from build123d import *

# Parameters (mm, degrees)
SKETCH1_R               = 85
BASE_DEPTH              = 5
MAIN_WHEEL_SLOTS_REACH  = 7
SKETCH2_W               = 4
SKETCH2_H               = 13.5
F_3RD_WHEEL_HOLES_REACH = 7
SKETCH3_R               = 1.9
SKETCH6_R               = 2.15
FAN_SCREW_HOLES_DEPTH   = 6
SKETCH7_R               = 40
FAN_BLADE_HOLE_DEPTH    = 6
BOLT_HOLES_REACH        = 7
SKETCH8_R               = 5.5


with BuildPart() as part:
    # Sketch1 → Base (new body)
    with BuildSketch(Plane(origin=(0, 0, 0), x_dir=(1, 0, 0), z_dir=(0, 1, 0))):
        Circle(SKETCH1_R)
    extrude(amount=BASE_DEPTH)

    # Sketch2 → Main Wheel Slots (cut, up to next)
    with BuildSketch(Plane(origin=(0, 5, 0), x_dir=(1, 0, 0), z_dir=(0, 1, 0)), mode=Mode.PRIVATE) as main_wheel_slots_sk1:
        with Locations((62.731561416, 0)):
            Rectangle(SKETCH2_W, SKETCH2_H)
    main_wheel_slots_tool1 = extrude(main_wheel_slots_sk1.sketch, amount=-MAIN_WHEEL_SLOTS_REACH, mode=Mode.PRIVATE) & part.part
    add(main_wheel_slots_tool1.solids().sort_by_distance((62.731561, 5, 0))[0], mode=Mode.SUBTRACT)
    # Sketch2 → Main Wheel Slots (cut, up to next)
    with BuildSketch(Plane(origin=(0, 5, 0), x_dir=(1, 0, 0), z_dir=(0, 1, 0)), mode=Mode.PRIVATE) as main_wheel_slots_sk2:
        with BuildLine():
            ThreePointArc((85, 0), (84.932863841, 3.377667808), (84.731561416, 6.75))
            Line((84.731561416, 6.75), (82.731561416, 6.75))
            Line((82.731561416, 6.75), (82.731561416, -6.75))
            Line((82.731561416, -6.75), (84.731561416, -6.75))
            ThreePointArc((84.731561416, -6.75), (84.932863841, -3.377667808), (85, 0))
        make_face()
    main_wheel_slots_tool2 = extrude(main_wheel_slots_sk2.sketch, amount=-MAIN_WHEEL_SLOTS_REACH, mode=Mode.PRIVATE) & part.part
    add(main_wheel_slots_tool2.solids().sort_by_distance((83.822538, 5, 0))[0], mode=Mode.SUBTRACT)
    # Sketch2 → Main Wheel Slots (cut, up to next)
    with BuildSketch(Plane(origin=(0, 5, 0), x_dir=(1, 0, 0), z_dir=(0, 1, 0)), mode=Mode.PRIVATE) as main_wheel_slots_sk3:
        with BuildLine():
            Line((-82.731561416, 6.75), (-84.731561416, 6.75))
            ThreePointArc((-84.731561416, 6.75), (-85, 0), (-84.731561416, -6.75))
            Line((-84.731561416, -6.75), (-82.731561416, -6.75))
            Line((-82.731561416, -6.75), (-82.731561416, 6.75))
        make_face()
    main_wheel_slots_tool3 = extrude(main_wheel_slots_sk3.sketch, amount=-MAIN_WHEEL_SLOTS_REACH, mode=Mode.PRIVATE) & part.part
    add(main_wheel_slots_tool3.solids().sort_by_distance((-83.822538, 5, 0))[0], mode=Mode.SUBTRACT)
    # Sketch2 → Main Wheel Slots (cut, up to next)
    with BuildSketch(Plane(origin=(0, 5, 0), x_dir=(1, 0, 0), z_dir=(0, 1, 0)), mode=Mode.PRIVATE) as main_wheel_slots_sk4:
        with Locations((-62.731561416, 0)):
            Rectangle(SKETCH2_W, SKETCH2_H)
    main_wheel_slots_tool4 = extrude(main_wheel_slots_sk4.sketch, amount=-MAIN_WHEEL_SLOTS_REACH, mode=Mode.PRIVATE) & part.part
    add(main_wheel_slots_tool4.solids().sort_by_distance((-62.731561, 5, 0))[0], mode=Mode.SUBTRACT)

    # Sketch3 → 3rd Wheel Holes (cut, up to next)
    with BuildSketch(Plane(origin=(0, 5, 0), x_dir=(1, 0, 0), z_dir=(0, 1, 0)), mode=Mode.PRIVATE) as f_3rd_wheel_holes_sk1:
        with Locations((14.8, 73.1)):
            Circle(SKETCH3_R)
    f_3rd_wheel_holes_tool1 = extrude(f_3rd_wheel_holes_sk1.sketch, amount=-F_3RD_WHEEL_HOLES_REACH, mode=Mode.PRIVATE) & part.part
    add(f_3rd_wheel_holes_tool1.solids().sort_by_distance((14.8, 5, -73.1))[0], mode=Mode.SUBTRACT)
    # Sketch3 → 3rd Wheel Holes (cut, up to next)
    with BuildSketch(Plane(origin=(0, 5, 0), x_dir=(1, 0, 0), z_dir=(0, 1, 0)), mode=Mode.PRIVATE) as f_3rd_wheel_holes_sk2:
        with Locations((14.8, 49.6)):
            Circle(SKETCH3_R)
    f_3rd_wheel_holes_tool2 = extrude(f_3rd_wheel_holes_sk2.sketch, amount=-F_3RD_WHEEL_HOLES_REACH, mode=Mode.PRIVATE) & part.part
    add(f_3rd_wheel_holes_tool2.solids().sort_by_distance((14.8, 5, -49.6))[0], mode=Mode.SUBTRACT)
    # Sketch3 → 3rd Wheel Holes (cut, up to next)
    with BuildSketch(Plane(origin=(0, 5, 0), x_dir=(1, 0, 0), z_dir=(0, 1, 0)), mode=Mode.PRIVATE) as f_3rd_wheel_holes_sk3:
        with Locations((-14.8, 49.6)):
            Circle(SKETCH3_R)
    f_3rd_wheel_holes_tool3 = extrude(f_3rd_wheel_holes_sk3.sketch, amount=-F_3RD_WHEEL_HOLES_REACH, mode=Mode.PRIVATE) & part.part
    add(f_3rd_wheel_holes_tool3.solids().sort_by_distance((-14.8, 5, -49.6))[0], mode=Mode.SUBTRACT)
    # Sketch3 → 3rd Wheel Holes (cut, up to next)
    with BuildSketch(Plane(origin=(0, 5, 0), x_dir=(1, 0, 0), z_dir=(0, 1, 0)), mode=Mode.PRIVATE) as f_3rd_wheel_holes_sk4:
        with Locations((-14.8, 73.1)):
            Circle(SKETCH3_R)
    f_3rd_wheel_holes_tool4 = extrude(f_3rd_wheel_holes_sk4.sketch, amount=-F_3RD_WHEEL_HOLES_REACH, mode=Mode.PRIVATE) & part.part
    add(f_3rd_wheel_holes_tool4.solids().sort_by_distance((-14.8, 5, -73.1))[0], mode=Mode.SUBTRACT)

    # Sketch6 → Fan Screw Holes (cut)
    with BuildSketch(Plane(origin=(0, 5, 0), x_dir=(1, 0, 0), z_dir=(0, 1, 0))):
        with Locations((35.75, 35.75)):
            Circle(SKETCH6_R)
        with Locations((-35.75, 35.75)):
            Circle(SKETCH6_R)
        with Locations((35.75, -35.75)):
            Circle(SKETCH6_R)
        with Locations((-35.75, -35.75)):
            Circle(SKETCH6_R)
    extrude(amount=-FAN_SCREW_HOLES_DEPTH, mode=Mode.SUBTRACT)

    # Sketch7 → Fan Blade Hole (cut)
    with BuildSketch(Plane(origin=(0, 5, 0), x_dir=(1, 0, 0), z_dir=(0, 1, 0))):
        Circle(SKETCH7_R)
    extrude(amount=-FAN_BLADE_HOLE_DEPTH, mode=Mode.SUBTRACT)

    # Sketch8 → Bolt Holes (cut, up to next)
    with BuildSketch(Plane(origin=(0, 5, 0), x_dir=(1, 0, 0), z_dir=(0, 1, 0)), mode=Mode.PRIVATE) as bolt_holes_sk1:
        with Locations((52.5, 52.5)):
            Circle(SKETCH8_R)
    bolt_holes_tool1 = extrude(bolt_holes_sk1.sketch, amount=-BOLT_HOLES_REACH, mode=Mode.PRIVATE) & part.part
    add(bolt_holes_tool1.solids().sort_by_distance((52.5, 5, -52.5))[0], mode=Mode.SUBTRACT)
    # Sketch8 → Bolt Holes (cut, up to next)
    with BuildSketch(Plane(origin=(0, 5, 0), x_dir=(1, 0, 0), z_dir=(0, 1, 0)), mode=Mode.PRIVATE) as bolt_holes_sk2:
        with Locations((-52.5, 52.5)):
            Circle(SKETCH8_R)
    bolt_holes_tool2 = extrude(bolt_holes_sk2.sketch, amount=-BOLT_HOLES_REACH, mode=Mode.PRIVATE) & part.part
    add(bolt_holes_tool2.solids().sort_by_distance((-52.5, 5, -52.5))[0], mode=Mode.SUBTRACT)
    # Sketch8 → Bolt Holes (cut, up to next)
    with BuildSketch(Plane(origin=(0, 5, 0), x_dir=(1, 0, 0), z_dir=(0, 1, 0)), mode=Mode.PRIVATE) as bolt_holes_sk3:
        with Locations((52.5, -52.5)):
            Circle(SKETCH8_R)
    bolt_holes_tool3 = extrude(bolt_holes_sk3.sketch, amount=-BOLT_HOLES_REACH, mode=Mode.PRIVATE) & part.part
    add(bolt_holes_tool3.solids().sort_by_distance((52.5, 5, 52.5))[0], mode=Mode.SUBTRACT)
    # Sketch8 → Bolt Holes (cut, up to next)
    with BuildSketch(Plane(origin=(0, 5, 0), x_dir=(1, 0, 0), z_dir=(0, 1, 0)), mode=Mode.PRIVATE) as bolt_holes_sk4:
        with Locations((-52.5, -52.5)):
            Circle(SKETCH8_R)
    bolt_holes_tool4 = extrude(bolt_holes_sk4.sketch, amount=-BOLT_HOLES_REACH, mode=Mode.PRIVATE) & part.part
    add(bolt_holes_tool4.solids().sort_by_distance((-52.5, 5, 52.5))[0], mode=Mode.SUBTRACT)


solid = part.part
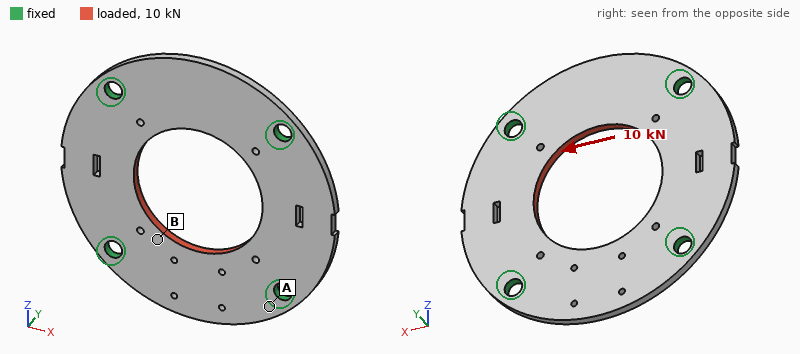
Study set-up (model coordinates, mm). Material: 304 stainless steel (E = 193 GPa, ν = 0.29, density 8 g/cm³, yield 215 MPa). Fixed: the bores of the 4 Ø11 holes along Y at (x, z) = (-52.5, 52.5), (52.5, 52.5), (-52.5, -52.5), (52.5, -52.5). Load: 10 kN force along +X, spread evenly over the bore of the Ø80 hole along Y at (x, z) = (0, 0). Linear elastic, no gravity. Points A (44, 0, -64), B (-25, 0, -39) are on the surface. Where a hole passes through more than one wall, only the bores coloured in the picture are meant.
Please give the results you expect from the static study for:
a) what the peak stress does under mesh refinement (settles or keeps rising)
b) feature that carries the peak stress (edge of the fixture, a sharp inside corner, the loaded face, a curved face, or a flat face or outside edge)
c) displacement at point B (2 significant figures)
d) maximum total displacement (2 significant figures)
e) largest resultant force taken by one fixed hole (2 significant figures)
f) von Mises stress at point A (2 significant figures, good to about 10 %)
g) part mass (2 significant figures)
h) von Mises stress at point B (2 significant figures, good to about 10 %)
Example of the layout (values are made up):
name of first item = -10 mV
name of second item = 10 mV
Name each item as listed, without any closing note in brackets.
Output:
what the peak stress does under mesh refinement = keeps rising
feature that carries the peak stress = edge of the fixture
displacement at point B = 2.5 µm
maximum total displacement = 5.7 µm
largest resultant force taken by one fixed hole = 2.5 kN
von Mises stress at point A = 5.9 MPa
part mass = 680 g
von Mises stress at point B = 15 MPa
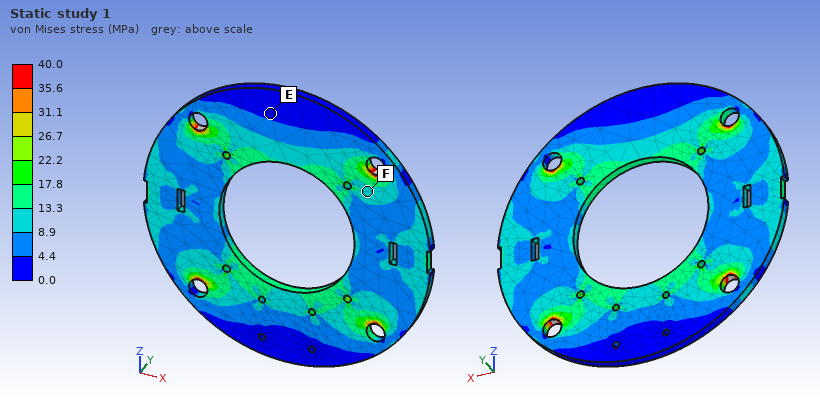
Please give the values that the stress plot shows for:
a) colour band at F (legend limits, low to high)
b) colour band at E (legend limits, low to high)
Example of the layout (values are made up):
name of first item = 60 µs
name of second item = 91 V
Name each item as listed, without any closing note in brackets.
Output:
colour band at F = 8.9 to 13.3 MPa
colour band at E = 0.0 to 4.4 MPa
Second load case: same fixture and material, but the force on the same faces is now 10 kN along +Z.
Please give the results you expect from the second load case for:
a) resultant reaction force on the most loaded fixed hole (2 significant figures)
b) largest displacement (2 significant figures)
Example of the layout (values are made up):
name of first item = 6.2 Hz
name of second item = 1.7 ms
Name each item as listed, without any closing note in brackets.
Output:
resultant reaction force on the most loaded fixed hole = 2.5 kN
largest displacement = 5.6 µm
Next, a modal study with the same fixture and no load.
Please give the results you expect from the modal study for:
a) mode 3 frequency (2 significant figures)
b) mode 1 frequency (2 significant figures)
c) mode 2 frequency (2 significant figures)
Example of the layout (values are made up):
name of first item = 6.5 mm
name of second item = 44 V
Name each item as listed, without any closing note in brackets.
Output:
mode 3 frequency = 2200 Hz
mode 1 frequency = 2000 Hz
mode 2 frequency = 2100 Hz
